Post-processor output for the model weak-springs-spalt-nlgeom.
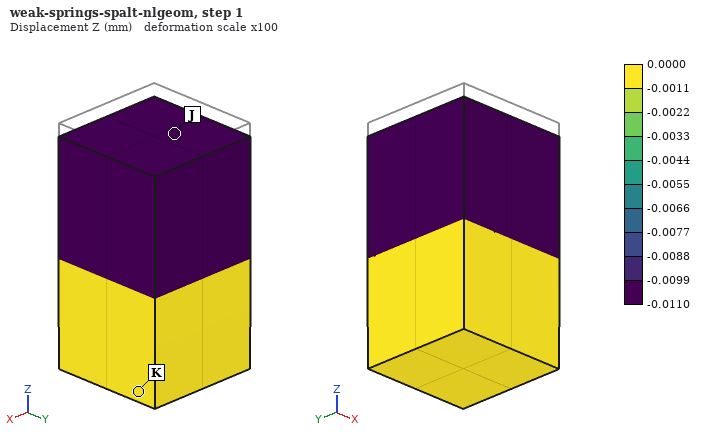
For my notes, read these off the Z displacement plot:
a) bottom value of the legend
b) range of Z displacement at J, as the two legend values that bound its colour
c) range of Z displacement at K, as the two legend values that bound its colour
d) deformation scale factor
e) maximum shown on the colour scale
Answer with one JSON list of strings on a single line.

["-0.0110 mm", "-0.0110 to -0.0099 mm", "-0.0011 to 0.0000 mm", "100", "0.0000 mm"]
